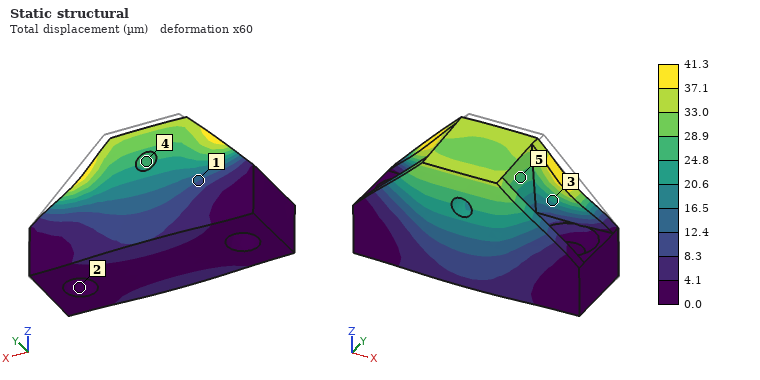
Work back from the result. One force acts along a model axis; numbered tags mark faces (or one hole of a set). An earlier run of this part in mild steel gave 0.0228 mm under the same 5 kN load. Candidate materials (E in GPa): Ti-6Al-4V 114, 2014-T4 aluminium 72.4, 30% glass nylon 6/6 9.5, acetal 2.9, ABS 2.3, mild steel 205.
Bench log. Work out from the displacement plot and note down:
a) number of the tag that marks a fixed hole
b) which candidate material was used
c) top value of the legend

2
Ti-6Al-4V
41.3 µm
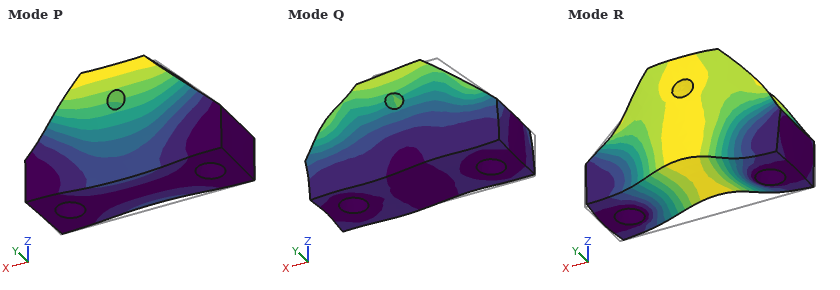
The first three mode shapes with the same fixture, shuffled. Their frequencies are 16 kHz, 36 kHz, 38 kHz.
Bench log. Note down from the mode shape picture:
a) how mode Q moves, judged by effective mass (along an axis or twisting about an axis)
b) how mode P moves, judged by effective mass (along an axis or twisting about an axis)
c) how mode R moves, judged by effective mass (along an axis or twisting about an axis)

along X
along Y
along Z
